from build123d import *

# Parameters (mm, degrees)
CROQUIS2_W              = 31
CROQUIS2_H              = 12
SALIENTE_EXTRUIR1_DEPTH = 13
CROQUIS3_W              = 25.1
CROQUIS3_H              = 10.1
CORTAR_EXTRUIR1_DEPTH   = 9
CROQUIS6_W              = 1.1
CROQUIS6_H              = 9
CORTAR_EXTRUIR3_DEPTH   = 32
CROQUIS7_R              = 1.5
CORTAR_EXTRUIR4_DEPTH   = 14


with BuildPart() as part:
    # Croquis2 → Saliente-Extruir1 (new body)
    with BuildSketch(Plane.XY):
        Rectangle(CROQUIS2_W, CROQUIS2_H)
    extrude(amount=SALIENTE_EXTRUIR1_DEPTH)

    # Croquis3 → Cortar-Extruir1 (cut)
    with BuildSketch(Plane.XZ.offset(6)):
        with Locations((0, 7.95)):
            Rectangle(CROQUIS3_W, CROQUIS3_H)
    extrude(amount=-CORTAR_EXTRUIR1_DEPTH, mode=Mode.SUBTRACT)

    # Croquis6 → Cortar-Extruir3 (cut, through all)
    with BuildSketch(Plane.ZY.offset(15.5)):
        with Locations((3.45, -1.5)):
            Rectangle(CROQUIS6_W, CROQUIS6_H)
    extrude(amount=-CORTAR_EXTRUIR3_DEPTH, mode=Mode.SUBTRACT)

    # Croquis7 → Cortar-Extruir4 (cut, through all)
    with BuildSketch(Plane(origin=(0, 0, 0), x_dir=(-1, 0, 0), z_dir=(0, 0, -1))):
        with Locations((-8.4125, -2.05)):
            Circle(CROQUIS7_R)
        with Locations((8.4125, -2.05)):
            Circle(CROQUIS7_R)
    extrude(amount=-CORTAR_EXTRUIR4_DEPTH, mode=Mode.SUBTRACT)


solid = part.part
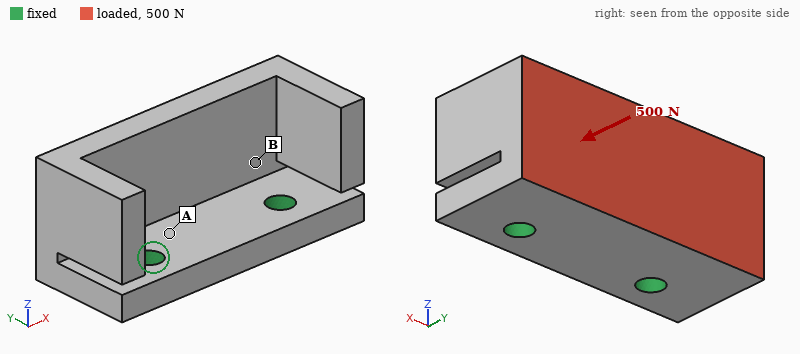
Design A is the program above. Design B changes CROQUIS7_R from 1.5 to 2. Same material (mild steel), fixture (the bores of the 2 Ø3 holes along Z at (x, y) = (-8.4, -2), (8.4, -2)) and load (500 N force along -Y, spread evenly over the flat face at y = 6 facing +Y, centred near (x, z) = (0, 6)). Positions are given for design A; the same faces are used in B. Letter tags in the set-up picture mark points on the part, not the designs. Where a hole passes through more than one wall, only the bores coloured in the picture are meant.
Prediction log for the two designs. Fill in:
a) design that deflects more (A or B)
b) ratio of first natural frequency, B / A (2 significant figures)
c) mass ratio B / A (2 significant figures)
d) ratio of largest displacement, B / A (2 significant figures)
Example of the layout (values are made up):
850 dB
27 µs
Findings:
A
1.1
0.99
0.91
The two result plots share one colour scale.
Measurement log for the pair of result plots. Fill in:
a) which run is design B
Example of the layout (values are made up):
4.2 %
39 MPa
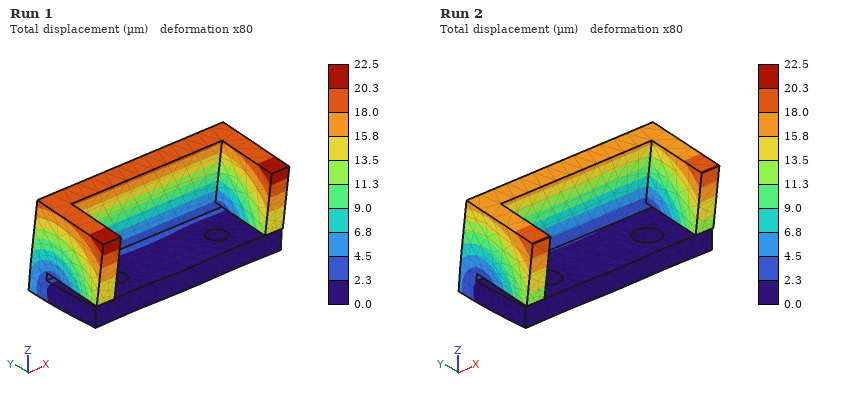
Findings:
Run 2
